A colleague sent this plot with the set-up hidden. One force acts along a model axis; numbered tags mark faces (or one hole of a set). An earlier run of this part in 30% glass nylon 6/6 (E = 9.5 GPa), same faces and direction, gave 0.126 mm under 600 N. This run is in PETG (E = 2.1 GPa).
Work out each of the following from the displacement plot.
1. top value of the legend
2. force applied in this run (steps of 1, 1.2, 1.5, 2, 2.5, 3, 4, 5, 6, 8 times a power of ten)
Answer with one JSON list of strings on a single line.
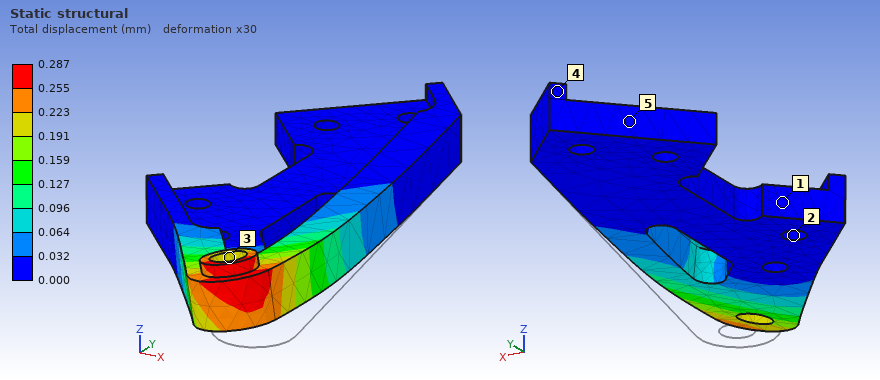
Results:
["0.287 mm", "300 N"]
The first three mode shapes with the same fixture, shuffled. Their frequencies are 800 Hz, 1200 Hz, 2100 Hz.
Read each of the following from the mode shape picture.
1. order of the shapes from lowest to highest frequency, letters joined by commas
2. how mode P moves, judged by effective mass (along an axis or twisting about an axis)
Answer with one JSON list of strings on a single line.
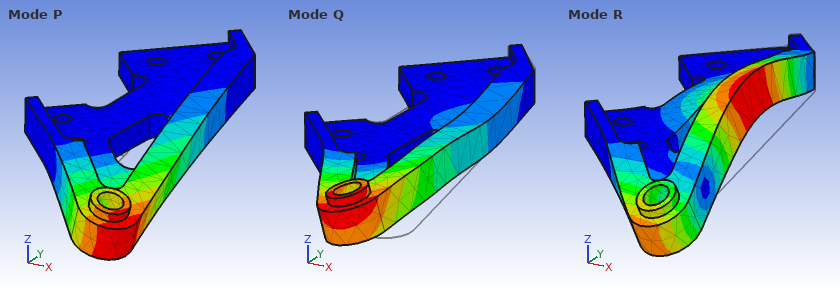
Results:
["P, R, Q", "along Z"]
